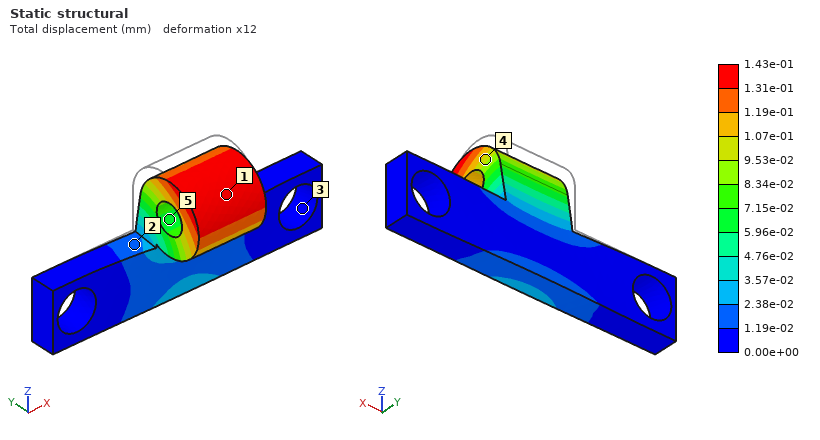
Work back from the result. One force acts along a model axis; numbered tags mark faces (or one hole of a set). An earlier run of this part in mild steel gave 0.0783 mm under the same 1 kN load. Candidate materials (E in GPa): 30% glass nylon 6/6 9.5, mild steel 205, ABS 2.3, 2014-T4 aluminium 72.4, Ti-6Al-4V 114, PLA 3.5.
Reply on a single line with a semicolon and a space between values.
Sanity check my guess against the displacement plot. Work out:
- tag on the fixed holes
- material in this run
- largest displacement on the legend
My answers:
3; Ti-6Al-4V; 1.43e-01 mm
